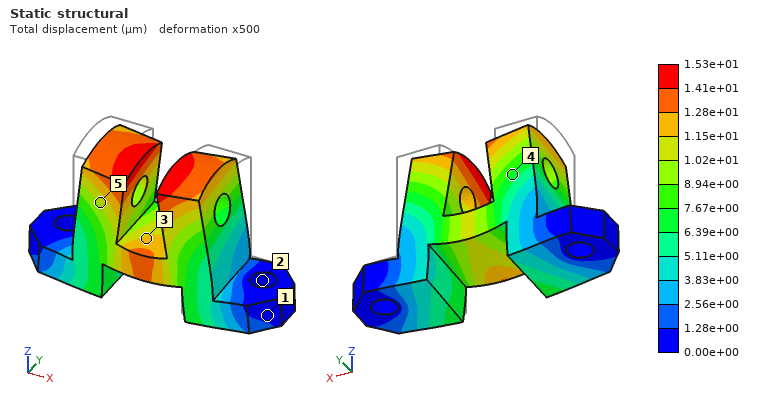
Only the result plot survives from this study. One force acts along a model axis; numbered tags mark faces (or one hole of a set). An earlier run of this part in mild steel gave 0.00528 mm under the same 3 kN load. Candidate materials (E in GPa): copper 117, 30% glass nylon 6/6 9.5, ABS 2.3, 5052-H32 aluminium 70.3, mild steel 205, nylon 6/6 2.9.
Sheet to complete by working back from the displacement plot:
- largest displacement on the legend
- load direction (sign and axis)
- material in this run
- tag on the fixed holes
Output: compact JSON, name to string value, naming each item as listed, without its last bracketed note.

{"largest displacement on the legend": "1.53e+01 µm", "load direction": "-Z", "material in this run": "5052-H32 aluminium", "tag on the fixed holes": "2"}
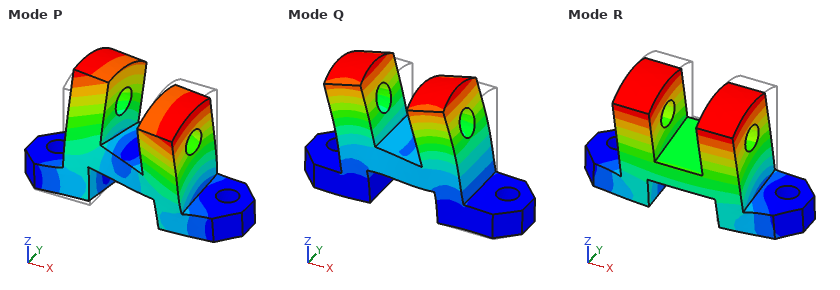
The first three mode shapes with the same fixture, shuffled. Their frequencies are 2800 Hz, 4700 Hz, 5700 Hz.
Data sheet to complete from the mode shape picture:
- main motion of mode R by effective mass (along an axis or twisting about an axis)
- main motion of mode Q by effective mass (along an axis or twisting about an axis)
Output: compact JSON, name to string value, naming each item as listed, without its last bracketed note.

{"main motion of mode R by effective mass": "along Y", "main motion of mode Q by effective mass": "along X"}
